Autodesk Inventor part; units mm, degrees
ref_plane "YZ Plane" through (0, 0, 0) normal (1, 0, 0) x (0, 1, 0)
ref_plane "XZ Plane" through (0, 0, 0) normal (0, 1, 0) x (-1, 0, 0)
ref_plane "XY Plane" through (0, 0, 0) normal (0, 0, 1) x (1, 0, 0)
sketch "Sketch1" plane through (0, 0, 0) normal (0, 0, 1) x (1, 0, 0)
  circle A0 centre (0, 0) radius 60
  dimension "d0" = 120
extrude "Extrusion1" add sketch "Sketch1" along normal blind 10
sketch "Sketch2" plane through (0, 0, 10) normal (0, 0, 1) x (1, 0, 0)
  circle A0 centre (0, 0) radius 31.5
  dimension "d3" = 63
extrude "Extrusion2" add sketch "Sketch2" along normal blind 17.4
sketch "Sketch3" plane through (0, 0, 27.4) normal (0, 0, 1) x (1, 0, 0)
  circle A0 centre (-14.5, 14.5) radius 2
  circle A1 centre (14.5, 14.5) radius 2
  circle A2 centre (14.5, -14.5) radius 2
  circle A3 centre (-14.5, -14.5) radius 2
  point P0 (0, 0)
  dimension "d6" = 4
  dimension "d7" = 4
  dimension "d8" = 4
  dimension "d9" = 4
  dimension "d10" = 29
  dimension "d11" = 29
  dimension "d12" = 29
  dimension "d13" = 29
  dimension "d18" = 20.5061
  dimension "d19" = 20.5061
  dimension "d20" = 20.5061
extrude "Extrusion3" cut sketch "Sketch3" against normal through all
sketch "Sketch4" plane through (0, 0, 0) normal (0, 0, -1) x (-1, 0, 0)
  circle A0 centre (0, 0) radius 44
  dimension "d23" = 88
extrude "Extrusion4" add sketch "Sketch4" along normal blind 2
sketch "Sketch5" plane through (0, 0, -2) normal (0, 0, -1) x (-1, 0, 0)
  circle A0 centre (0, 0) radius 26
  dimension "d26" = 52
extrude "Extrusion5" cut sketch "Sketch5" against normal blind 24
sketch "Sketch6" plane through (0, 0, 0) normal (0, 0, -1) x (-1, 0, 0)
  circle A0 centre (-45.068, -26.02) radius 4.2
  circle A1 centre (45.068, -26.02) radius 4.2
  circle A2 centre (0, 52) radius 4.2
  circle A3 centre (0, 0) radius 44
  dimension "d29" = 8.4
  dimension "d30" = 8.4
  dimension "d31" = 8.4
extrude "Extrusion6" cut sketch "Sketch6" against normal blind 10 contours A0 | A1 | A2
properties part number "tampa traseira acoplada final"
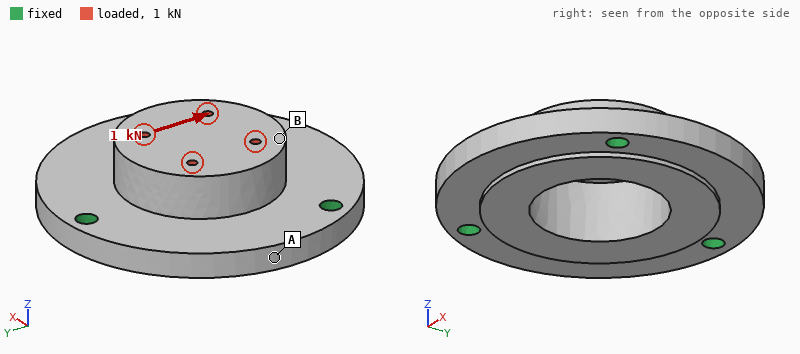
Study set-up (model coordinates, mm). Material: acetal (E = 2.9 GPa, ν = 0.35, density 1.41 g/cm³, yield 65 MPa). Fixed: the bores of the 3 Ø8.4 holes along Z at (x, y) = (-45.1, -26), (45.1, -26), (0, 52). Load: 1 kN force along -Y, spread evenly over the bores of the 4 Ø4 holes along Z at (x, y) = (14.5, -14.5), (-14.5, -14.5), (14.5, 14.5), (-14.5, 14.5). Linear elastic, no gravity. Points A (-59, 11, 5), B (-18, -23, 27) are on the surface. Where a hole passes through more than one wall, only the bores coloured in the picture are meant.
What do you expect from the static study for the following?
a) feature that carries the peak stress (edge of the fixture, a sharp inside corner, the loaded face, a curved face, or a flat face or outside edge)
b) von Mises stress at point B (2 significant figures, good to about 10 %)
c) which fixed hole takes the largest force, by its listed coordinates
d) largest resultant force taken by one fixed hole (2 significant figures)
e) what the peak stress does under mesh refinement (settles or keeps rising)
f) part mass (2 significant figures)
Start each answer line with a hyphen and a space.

- edge of the fixture
- 2.4 MPa
- (0, 52)
- 420 N
- keeps rising
- 180 g
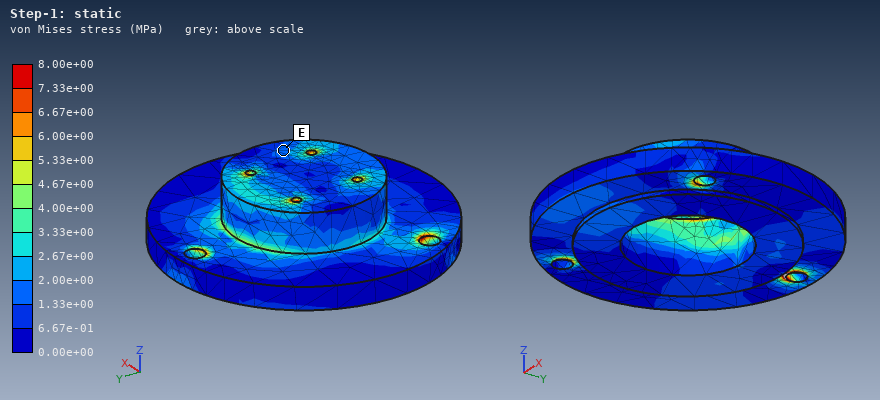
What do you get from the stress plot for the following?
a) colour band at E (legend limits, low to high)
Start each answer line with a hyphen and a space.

- 1.33e+00 to 2.00e+00 MPa
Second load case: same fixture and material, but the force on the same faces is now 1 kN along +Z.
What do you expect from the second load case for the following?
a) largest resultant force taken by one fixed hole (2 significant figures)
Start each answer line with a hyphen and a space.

- 340 N
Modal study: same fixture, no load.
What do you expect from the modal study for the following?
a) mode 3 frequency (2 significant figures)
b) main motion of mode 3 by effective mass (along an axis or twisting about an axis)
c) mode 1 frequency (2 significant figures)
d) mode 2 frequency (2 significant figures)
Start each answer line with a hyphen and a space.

- 1500 Hz
- along Z
- 1400 Hz
- 1400 Hz
